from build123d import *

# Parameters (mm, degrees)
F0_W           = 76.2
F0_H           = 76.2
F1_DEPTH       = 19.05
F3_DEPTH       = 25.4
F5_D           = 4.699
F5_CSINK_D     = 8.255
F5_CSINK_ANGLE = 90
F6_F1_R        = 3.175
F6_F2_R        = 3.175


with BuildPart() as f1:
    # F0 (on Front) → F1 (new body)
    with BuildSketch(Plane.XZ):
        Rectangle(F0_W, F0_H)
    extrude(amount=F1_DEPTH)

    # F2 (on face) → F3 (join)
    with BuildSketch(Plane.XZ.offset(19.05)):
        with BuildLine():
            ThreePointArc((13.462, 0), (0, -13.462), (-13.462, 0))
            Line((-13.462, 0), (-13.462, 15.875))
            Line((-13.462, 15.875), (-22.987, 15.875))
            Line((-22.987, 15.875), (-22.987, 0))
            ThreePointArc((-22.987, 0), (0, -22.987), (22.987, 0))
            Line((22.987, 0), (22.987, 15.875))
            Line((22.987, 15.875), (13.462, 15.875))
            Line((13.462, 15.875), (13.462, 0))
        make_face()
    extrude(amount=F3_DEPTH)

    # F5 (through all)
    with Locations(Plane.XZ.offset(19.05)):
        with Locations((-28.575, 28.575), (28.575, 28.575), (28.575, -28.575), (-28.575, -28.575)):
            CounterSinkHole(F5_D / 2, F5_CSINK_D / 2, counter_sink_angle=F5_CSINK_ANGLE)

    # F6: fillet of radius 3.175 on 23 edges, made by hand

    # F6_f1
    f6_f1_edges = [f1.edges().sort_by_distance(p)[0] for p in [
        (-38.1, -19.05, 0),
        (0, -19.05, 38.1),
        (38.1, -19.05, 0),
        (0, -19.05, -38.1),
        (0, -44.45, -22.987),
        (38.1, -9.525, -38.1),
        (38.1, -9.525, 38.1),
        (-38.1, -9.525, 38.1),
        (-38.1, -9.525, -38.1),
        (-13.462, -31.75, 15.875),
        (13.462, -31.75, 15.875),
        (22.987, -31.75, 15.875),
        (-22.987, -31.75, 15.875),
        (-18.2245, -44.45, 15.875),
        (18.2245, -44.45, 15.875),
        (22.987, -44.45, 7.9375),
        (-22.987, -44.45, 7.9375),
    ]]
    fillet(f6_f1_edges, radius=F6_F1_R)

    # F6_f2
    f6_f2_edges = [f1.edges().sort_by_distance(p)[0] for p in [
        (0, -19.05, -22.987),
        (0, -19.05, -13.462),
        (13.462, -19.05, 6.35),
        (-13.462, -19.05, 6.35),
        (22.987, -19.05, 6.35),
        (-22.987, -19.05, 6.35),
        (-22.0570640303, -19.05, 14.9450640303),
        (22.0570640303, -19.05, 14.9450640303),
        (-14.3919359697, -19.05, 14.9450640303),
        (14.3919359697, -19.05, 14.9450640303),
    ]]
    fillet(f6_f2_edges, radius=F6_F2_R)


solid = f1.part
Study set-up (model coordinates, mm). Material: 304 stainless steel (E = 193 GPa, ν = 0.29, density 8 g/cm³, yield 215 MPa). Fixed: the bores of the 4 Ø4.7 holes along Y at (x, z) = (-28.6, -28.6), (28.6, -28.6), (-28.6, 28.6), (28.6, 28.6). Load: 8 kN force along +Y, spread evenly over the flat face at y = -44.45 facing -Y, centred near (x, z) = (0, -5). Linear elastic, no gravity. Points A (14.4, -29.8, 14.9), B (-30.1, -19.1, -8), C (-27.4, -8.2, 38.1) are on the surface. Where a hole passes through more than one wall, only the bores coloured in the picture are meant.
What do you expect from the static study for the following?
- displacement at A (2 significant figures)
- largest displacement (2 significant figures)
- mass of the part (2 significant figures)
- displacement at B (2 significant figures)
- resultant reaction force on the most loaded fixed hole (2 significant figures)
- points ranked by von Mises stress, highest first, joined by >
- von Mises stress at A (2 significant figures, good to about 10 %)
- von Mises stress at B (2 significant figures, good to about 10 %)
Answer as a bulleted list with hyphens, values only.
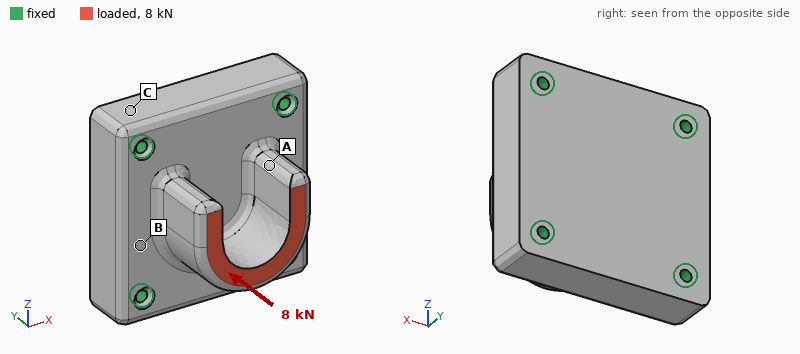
- 2.8 µm
- 4.5 µm
- 1.0 kg
- 1.6 µm
- 2.4 kN
- A > B > C
- 11 MPa
- 5.6 MPa
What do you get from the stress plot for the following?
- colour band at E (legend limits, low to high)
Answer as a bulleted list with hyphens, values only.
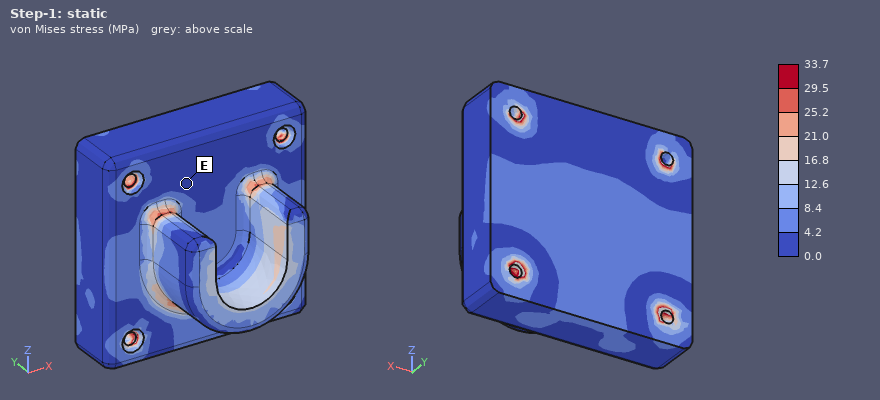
- 0.0 to 4.2 MPa
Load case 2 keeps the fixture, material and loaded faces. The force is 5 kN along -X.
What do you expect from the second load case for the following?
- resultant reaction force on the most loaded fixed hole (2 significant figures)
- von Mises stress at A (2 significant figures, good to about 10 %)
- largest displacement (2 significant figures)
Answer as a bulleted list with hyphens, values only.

- 2.7 kN
- 35 MPa
- 20 µm
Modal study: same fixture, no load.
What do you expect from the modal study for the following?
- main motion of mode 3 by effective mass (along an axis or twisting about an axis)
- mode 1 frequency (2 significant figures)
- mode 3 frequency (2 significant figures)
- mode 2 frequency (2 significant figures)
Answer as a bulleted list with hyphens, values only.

- along Z
- 11 kHz
- 13 kHz
- 11 kHz
